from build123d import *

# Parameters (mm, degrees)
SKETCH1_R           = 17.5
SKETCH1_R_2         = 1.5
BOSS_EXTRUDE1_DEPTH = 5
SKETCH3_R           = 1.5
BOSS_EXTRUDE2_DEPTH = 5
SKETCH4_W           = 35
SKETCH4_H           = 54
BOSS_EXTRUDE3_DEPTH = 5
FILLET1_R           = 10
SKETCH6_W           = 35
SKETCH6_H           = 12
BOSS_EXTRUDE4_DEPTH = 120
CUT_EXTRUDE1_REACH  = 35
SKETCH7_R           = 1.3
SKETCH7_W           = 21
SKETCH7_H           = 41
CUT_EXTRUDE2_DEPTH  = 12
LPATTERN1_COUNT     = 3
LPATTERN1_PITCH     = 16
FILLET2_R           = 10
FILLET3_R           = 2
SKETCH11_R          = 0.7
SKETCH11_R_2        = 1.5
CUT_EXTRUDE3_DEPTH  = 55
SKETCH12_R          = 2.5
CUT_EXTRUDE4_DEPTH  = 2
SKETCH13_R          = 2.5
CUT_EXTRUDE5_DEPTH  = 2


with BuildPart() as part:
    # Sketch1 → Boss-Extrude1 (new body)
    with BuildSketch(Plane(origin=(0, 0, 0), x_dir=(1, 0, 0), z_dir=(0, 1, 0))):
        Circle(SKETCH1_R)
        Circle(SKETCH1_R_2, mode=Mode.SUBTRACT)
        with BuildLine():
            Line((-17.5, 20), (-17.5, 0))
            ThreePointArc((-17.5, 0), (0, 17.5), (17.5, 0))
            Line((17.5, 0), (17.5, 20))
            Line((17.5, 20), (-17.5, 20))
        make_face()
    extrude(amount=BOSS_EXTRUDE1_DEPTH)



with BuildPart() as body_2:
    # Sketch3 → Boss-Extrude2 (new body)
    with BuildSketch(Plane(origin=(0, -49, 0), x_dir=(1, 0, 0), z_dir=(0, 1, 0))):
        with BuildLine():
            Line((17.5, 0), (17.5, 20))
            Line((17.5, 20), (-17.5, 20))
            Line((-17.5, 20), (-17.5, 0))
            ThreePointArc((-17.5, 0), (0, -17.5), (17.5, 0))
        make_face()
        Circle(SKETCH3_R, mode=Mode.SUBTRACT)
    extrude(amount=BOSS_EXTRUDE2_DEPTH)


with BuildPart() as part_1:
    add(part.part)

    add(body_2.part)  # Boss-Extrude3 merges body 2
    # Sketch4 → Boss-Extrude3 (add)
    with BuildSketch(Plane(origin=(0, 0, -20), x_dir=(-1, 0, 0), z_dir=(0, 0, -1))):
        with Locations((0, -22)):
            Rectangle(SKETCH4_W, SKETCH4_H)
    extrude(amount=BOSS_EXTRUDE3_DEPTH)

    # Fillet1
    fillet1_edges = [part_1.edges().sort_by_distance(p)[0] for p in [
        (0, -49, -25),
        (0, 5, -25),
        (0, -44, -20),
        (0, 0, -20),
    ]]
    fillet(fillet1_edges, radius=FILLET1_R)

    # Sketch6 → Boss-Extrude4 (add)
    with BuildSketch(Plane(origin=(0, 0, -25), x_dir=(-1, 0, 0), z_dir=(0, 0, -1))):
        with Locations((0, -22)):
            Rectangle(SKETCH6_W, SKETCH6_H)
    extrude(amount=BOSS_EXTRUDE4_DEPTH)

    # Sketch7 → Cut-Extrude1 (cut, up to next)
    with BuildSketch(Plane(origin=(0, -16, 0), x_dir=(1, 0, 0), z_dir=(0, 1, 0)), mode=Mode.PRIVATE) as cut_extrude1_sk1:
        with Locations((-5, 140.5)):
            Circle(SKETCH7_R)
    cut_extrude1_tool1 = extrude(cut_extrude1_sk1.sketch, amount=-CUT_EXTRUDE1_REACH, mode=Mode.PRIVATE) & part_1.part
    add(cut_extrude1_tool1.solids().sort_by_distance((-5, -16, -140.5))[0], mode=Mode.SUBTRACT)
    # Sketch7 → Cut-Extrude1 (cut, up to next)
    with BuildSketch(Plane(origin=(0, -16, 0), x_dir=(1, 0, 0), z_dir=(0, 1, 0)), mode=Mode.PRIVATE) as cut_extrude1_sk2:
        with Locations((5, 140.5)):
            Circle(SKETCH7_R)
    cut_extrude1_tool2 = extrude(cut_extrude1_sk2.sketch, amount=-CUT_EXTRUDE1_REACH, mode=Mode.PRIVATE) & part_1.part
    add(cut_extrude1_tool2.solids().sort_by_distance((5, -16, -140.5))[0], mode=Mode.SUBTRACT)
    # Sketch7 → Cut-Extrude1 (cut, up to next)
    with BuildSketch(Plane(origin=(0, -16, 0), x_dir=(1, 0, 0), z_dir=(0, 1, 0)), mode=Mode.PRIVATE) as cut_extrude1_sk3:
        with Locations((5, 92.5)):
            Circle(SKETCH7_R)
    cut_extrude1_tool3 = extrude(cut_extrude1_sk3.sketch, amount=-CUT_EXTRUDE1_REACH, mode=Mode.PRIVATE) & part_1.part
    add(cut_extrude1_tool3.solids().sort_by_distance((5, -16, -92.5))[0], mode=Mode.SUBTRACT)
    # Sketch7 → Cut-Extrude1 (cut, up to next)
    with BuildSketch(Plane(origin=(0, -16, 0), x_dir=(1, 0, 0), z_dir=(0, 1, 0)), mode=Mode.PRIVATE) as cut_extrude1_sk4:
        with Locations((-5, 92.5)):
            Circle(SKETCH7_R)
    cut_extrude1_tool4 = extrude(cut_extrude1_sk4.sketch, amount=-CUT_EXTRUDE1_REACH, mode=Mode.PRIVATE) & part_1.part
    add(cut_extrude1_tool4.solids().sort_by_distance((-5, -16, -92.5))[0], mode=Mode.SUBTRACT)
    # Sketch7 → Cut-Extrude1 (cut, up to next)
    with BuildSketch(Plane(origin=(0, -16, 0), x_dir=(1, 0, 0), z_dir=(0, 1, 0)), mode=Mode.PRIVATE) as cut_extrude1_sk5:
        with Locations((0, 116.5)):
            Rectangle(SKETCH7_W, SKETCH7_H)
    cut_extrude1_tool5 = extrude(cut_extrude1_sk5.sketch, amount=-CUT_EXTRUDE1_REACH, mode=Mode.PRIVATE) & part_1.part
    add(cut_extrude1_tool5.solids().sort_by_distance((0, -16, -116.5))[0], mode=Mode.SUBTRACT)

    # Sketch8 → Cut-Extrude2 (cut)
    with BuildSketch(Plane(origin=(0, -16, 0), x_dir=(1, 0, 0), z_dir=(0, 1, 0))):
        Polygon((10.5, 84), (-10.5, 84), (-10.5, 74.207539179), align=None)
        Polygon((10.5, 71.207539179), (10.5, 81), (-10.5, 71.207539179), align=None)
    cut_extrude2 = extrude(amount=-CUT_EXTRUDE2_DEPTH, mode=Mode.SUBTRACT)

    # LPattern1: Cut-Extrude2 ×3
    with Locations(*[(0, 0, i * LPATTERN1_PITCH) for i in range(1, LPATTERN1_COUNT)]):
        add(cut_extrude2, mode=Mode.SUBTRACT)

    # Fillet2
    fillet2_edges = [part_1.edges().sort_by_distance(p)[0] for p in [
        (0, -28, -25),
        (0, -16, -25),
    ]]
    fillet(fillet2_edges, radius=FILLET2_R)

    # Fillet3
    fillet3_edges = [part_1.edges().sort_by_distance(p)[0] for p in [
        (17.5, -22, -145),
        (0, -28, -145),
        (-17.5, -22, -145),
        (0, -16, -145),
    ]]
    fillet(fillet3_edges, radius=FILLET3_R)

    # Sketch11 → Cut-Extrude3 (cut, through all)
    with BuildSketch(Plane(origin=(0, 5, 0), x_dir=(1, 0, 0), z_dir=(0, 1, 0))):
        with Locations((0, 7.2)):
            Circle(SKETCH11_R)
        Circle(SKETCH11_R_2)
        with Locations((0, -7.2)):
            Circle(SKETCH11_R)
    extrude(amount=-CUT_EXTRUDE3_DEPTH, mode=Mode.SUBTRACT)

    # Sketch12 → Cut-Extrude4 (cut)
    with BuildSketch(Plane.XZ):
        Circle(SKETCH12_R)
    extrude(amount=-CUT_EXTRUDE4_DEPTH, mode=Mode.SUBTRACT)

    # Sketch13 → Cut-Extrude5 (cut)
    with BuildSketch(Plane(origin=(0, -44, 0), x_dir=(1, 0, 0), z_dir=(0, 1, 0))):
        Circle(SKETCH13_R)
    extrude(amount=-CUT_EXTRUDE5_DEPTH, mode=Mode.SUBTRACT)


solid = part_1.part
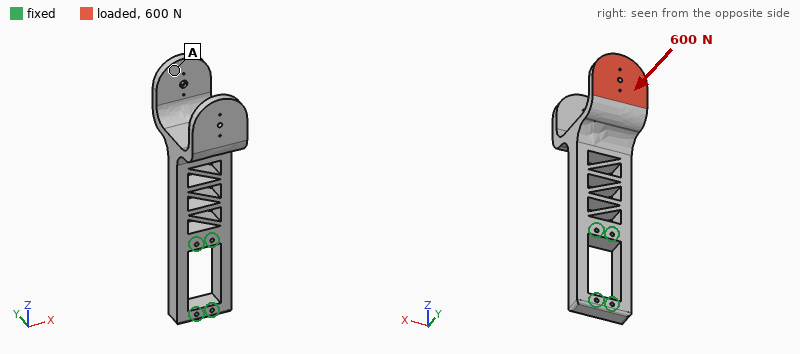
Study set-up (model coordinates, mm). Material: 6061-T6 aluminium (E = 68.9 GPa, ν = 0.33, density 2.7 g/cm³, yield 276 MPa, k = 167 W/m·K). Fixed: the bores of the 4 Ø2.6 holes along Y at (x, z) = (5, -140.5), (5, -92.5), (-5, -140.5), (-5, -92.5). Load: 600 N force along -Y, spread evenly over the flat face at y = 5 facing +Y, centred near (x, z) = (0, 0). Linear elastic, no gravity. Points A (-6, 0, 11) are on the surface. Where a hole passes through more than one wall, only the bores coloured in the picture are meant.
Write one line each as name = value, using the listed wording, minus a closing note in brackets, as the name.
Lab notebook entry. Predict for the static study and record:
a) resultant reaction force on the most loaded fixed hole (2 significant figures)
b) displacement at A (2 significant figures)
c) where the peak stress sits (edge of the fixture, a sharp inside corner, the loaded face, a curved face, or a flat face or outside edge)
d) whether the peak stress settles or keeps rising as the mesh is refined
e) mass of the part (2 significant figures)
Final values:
resultant reaction force on the most loaded fixed hole = 500 N
displacement at A = 1.5 mm
where the peak stress sits = edge of the fixture
whether the peak stress settles or keeps rising as the mesh is refined = keeps rising
mass of the part = 150 g
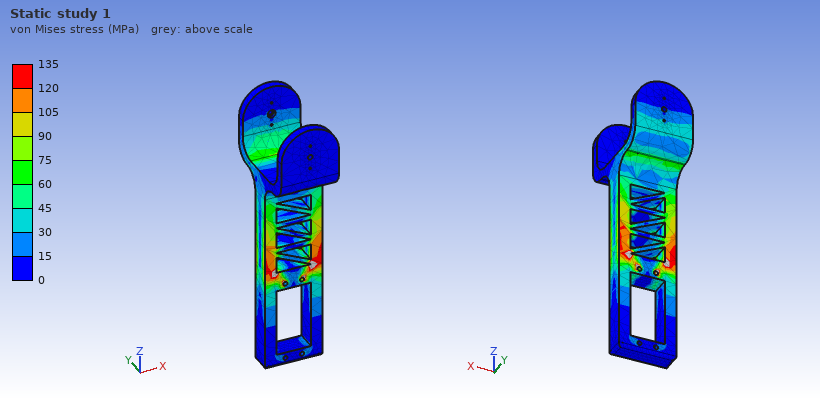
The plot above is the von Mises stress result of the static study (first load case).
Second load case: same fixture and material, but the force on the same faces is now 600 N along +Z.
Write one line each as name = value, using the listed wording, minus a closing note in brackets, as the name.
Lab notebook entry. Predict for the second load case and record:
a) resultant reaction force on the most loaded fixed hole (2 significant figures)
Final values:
resultant reaction force on the most loaded fixed hole = 280 N
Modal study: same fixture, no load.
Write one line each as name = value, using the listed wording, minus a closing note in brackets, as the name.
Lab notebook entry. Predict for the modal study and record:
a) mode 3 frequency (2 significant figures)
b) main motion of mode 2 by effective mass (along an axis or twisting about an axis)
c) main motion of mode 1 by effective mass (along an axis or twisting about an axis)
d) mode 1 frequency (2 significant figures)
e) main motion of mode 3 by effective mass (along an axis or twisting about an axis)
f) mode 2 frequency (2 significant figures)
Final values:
mode 3 frequency = 1400 Hz
main motion of mode 2 by effective mass = along X
main motion of mode 1 by effective mass = along Y
mode 1 frequency = 500 Hz
main motion of mode 3 by effective mass = twisting about Z
mode 2 frequency = 1200 Hz
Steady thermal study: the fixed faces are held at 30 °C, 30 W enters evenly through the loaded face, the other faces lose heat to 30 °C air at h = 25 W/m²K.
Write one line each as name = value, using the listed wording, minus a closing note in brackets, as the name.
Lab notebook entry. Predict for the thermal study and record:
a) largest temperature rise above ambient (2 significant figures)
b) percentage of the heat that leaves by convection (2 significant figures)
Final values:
largest temperature rise above ambient = 68 K
percentage of the heat that leaves by convection = 43 %
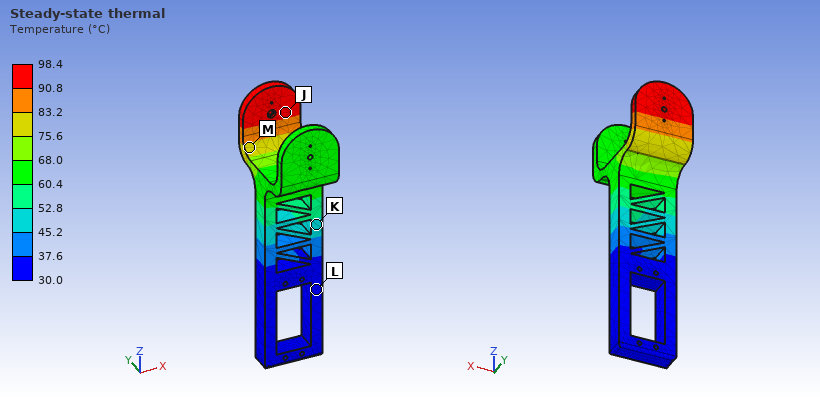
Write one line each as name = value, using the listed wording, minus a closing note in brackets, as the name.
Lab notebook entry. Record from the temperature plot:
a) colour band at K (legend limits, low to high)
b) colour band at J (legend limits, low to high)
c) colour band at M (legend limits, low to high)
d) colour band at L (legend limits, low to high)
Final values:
colour band at K = 45.2 to 52.8 °C
colour band at J = 90.8 to 98.4 °C
colour band at M = 75.6 to 83.2 °C
colour band at L = 30.0 to 37.6 °C
